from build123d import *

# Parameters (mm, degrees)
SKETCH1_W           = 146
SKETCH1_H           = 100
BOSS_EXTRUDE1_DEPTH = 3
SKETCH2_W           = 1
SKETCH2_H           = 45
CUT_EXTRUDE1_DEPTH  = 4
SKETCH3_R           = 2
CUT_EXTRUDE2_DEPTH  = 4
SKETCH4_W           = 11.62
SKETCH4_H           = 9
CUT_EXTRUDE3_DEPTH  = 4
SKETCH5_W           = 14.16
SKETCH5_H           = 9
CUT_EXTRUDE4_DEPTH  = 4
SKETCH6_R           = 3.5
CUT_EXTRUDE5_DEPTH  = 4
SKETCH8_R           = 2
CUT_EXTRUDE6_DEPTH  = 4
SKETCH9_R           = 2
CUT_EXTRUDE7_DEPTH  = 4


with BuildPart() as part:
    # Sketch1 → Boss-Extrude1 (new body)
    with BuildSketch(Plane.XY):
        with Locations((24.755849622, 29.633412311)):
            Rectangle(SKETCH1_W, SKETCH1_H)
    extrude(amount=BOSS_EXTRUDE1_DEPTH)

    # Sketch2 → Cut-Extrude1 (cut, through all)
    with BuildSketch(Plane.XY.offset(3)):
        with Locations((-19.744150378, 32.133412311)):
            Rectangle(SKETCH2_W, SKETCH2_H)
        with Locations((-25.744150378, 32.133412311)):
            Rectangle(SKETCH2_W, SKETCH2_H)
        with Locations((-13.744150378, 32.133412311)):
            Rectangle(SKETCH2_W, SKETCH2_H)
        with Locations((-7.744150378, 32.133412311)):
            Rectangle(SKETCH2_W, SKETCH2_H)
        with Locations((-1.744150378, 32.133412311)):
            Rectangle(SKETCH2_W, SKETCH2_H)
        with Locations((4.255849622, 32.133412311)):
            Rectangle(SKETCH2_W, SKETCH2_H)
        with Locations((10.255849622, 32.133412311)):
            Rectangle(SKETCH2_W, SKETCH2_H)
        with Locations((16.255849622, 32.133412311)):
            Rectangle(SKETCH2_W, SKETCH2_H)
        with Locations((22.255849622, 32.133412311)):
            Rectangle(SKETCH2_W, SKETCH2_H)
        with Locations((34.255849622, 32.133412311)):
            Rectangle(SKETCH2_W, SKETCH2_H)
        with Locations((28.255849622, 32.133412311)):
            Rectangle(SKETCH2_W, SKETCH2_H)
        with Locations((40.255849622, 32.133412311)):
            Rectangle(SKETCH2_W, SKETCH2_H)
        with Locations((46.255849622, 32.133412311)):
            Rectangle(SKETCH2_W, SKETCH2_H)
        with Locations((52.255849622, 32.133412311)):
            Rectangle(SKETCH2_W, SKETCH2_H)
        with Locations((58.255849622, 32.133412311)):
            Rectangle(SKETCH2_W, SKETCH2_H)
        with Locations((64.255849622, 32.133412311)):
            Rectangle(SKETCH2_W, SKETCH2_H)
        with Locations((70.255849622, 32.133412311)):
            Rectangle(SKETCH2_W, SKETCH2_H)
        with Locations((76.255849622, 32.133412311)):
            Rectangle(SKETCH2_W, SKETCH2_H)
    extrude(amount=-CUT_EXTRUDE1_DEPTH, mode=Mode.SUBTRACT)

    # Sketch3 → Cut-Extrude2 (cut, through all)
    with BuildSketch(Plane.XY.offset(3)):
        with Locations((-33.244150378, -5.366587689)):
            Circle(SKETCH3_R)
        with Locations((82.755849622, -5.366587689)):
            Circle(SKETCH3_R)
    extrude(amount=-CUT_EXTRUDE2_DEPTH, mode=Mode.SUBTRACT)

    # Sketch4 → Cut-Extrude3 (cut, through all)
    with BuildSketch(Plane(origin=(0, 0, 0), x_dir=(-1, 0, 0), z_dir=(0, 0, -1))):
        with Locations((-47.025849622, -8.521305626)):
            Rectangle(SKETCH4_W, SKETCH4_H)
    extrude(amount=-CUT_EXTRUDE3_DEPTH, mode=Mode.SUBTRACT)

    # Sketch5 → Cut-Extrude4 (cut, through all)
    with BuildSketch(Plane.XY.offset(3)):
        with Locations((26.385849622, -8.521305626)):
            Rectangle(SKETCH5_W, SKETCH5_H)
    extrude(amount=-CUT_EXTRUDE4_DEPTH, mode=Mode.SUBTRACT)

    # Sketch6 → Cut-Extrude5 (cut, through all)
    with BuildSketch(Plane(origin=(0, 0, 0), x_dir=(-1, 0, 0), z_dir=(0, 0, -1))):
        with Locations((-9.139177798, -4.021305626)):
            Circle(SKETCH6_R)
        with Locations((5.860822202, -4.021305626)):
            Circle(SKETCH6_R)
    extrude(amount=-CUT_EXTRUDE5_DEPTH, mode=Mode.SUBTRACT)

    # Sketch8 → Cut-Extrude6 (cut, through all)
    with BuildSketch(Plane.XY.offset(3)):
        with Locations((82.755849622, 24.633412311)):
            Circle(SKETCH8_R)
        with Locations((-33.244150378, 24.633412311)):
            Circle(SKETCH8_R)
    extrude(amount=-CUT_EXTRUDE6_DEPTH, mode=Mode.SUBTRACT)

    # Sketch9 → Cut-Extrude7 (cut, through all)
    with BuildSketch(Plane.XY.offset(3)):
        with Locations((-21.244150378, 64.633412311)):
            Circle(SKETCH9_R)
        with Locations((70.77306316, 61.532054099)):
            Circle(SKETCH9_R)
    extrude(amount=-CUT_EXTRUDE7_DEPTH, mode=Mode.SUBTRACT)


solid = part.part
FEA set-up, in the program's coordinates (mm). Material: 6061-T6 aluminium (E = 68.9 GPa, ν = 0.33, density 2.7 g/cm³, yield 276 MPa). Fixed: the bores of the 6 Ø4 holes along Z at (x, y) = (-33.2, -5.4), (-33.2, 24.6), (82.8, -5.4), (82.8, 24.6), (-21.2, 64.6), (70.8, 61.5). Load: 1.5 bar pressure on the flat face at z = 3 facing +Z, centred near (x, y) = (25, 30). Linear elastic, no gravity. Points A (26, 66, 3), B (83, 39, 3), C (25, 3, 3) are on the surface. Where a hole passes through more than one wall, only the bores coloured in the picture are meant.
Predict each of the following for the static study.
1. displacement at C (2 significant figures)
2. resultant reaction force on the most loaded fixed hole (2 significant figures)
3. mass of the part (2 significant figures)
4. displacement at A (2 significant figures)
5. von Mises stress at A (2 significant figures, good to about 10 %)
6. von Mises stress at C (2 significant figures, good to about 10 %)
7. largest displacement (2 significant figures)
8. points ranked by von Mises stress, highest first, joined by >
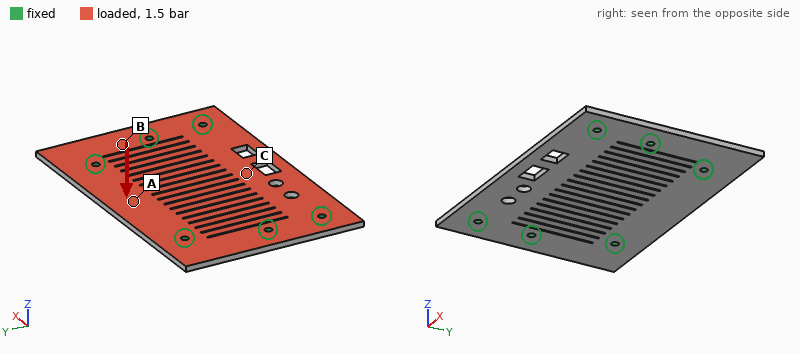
0.64 mm
490 N
110 g
0.34 mm
65 MPa
83 MPa
0.66 mm
C > A > B
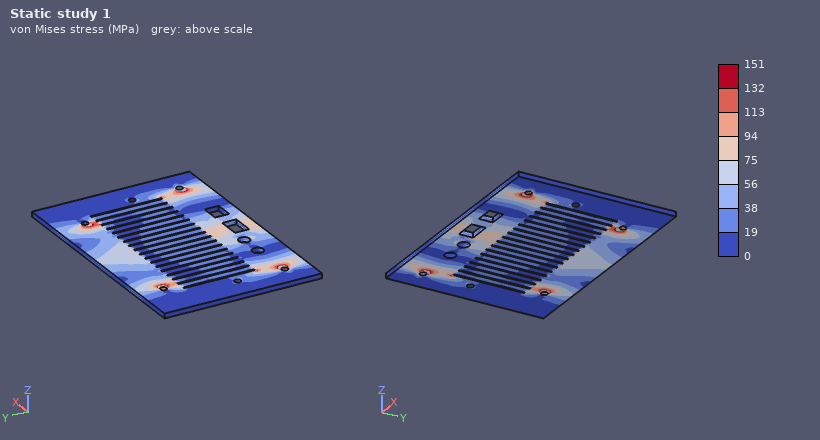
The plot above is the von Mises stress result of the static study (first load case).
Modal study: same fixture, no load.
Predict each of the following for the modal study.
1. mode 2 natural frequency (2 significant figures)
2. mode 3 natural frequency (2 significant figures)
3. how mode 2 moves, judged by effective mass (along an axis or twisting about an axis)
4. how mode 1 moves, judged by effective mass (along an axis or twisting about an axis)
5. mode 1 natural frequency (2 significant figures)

1700 Hz
2300 Hz
twisting about X
along Z
1000 Hz
